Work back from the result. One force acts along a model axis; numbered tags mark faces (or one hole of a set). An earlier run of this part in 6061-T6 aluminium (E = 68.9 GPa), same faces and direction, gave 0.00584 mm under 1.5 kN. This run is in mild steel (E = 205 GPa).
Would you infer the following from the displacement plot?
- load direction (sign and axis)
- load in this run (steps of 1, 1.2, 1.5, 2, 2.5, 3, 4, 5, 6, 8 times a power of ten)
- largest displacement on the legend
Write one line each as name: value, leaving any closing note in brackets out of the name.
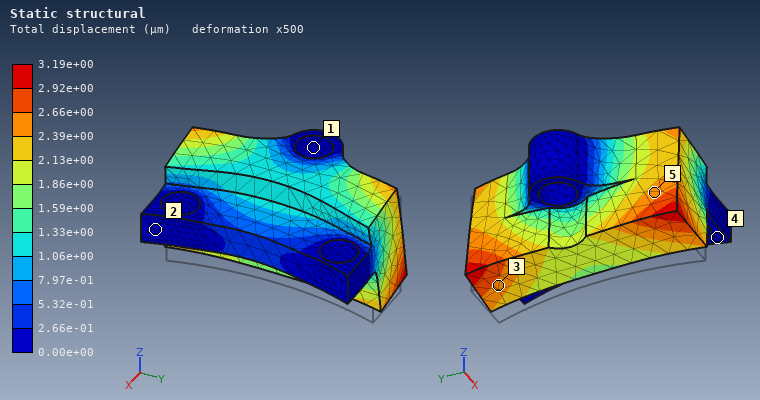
load direction: +Z
load in this run: 2.5 kN
largest displacement on the legend: 3.19e+00 µm
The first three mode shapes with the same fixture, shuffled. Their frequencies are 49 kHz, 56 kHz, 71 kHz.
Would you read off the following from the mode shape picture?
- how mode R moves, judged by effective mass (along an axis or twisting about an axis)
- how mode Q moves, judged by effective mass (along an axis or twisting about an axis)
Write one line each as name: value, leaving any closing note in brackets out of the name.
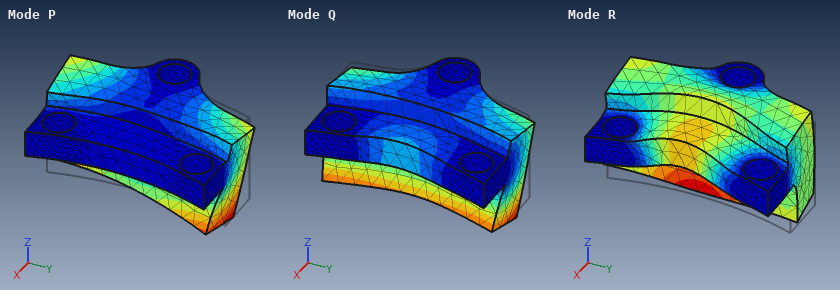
how mode R moves, judged by effective mass: along Z
how mode Q moves, judged by effective mass: along X
